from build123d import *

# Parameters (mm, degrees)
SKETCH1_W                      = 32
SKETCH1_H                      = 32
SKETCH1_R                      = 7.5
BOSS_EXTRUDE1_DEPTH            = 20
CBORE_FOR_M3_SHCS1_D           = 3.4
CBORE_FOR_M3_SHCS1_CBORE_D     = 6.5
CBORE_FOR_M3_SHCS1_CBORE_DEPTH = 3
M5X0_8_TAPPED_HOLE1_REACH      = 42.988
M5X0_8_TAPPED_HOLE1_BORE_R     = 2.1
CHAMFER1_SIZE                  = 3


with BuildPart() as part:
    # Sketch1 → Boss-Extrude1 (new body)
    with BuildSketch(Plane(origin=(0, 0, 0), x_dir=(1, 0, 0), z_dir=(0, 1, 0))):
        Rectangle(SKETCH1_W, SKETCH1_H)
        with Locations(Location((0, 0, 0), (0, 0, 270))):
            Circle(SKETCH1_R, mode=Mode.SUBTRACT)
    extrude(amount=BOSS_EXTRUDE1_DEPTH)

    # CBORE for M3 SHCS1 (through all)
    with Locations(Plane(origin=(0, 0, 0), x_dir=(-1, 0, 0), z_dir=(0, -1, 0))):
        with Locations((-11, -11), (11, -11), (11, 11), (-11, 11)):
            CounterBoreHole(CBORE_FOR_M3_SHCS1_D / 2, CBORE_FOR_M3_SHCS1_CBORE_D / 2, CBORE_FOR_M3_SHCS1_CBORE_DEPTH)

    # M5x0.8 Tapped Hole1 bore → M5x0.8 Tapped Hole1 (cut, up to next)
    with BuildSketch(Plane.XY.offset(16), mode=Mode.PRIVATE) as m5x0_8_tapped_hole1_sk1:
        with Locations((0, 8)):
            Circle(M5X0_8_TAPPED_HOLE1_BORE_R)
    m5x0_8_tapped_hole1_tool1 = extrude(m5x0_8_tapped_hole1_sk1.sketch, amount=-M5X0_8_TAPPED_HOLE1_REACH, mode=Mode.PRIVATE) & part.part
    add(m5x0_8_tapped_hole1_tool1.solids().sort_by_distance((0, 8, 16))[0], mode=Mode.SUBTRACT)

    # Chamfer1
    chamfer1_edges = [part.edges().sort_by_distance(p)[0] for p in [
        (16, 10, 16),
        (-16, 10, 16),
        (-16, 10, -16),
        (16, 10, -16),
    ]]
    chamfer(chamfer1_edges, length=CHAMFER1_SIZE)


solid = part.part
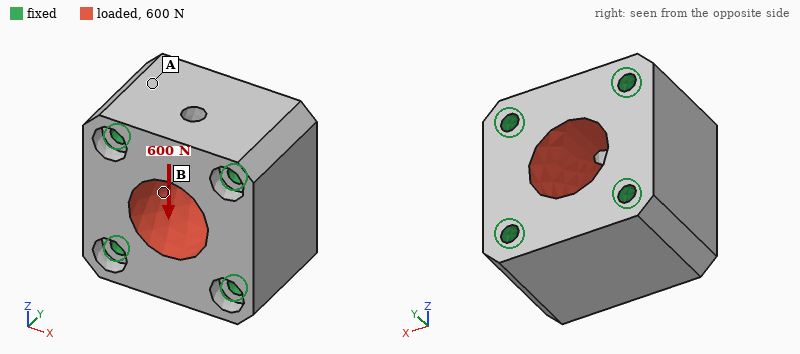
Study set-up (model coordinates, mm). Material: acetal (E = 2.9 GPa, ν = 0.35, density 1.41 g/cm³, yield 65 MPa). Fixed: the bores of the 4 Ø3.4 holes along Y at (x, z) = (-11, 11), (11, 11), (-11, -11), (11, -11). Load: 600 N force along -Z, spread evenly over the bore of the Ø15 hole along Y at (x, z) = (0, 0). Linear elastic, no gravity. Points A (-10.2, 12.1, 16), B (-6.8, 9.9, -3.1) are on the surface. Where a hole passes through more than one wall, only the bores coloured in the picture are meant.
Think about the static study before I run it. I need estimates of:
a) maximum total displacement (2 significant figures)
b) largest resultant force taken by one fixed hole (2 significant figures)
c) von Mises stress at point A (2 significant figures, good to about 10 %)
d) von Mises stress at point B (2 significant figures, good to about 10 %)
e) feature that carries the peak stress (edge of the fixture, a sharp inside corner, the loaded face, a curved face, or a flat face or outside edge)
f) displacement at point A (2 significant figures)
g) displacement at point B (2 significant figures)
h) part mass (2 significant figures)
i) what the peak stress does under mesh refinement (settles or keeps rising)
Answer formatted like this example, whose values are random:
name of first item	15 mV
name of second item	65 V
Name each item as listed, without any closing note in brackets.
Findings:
maximum total displacement	6.8 µm
largest resultant force taken by one fixed hole	160 N
von Mises stress at point A	0.48 MPa
von Mises stress at point B	1.3 MPa
feature that carries the peak stress	edge of the fixture
displacement at point A	1.2 µm
displacement at point B	3.0 µm
part mass	22 g
what the peak stress does under mesh refinement	keeps rising
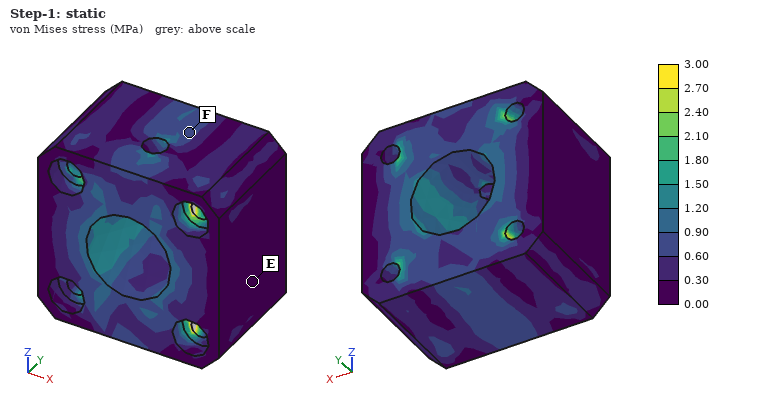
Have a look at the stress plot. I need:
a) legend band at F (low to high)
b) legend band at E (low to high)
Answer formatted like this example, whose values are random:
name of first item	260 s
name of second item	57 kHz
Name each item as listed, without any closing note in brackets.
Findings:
legend band at F	0.60 to 0.90 MPa
legend band at E	0.00 to 0.30 MPa
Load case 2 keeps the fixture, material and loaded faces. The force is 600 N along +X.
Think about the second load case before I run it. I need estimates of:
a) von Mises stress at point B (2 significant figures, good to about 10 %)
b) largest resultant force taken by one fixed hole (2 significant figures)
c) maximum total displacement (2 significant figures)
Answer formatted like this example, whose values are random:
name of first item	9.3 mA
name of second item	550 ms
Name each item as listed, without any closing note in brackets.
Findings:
von Mises stress at point B	0.54 MPa
largest resultant force taken by one fixed hole	160 N
maximum total displacement	6.9 µm
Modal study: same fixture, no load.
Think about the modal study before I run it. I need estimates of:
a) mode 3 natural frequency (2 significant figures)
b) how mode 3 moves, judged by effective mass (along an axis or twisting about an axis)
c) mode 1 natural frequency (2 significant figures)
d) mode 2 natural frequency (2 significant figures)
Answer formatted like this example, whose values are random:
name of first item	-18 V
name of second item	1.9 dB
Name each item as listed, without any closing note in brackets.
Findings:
mode 3 natural frequency	17 kHz
how mode 3 moves, judged by effective mass	along X
mode 1 natural frequency	13 kHz
mode 2 natural frequency	16 kHz
